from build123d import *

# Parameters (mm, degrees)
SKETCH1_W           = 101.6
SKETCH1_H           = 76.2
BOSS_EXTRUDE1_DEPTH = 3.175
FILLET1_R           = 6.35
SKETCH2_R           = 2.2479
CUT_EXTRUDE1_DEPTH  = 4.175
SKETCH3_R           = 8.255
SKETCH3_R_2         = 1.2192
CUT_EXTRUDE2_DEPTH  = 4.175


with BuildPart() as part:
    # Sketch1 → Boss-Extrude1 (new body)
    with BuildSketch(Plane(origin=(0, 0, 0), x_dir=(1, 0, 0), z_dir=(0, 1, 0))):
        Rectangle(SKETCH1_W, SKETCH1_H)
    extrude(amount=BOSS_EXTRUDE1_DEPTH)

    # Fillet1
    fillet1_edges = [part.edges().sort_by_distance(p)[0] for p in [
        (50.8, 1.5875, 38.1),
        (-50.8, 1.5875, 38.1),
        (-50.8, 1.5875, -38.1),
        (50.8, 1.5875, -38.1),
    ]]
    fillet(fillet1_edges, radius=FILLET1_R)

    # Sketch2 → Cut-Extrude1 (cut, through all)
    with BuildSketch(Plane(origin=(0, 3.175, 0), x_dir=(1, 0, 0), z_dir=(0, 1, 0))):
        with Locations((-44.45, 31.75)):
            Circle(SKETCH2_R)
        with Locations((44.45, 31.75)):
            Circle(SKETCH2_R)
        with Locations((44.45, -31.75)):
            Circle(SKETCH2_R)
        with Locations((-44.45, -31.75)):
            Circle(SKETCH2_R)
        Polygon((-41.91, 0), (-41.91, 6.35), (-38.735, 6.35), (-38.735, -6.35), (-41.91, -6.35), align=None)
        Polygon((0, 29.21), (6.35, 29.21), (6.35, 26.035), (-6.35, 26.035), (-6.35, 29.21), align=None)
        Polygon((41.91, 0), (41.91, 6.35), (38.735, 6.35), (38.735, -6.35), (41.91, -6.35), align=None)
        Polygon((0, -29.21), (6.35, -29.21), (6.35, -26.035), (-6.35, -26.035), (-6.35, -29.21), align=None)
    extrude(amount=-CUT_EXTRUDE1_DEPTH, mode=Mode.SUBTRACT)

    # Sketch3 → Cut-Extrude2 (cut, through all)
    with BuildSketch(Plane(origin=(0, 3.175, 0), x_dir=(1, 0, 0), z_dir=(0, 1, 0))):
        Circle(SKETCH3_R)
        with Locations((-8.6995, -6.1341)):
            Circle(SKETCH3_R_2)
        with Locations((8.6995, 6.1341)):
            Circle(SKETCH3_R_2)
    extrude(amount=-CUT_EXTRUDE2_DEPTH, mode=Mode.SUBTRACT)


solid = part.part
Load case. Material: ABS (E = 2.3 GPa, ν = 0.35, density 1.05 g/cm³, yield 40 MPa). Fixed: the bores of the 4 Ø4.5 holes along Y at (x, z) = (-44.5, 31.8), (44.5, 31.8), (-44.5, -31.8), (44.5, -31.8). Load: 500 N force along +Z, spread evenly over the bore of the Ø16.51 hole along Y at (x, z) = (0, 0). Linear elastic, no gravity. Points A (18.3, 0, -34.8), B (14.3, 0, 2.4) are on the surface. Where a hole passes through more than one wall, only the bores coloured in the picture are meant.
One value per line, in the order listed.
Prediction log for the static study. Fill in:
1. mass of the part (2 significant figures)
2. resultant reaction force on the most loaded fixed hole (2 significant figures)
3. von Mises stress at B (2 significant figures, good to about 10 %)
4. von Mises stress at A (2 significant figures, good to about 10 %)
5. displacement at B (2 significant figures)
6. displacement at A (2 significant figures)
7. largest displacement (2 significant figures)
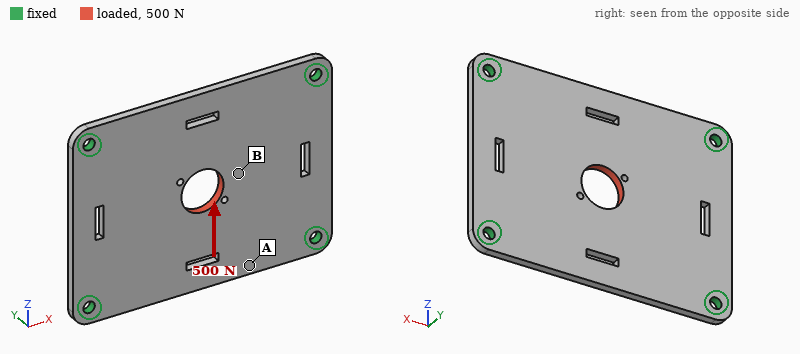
24 g
150 N
2.9 MPa
0.94 MPa
60 µm
52 µm
83 µm
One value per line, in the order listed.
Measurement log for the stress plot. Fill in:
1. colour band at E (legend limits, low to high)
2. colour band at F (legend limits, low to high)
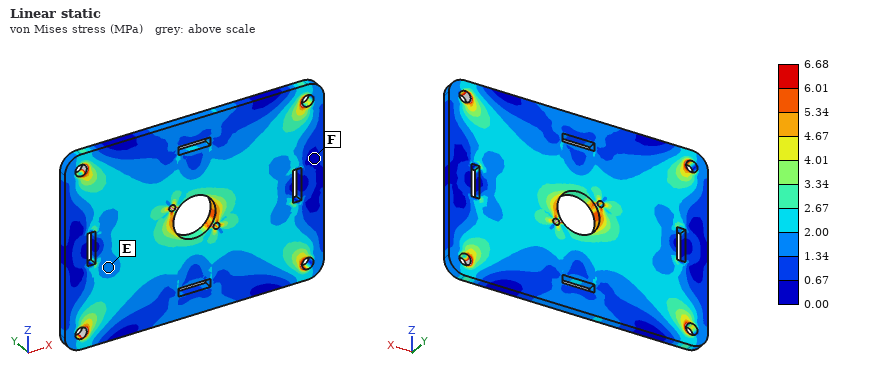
1.34 to 2.00 MPa
0.00 to 0.67 MPa
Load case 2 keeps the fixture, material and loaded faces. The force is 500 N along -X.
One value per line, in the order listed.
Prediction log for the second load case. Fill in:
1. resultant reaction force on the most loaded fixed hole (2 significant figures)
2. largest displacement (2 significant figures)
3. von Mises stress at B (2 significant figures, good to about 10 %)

140 N
58 µm
2.4 MPa
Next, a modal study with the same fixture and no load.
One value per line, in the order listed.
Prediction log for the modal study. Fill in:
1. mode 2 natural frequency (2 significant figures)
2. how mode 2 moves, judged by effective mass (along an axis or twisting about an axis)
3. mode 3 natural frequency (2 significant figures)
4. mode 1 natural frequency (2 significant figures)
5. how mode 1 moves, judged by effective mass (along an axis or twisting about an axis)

780 Hz
twisting about X
1100 Hz
500 Hz
along Y
